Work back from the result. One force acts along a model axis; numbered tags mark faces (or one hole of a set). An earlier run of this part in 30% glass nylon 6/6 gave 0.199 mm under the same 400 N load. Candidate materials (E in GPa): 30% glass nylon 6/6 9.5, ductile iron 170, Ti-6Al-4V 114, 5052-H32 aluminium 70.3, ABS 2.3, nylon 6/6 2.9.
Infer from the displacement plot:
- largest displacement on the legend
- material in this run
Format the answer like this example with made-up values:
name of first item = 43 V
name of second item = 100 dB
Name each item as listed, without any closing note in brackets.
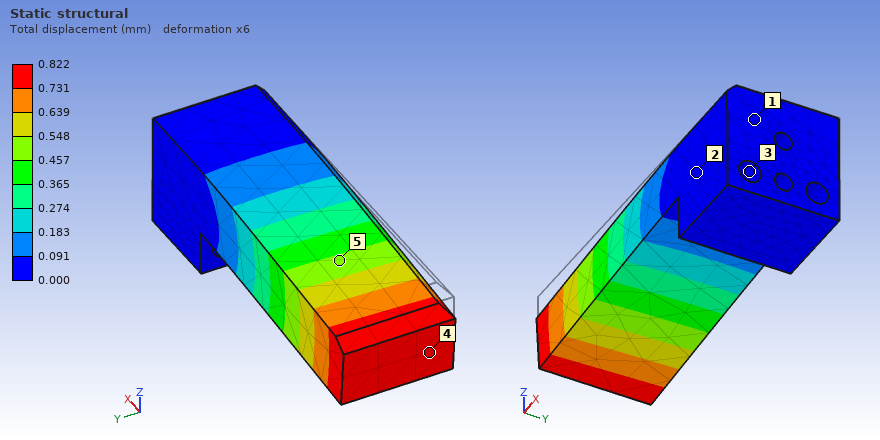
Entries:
largest displacement on the legend = 0.822 mm
material in this run = ABS
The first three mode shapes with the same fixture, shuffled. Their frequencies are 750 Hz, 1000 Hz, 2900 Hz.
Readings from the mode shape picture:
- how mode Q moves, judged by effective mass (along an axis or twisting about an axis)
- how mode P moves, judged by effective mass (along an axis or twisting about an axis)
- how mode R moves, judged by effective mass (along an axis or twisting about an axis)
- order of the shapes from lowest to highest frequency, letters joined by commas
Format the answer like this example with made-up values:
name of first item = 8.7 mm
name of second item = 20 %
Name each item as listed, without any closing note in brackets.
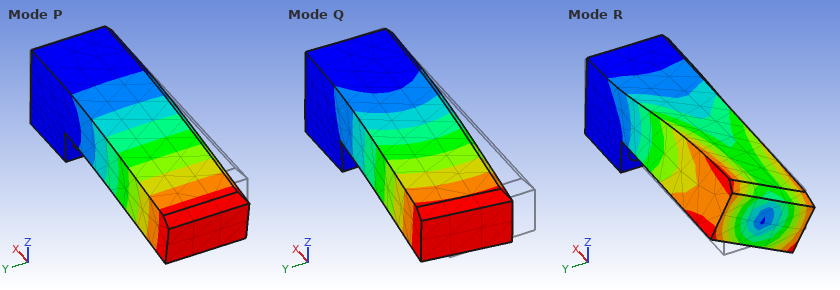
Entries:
how mode Q moves, judged by effective mass = along Y
how mode P moves, judged by effective mass = along Z
how mode R moves, judged by effective mass = twisting about X
order of the shapes from lowest to highest frequency, letters joined by commas = P, Q, R
